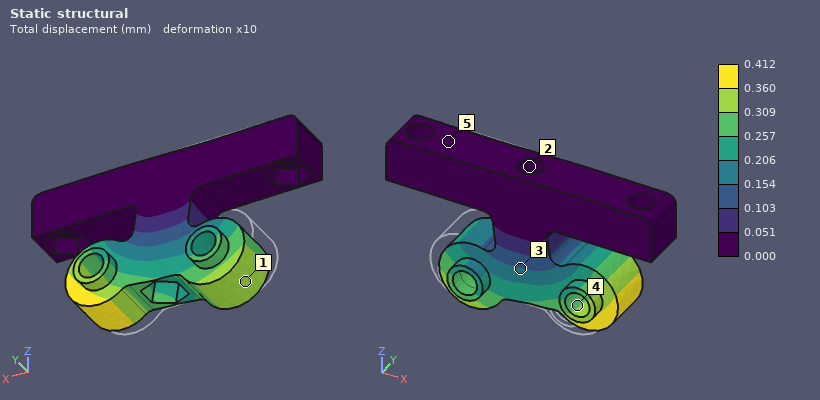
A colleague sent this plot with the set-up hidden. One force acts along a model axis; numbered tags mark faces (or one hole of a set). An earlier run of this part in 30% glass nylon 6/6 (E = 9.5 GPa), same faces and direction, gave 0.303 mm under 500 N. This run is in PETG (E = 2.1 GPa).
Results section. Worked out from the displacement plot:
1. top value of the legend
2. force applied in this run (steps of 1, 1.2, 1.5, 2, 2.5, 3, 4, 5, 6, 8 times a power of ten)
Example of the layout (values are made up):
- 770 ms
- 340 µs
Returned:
- 0.412 mm
- 150 N
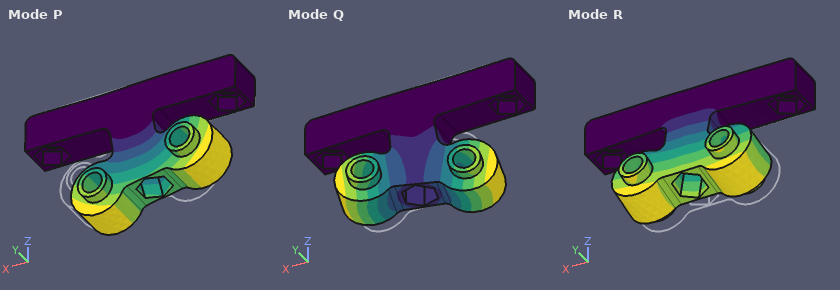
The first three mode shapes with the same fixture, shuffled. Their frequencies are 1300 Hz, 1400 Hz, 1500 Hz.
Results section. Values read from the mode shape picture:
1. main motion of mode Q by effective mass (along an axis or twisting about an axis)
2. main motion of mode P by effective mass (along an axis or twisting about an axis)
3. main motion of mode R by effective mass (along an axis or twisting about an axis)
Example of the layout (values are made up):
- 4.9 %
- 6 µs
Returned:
- twisting about Z
- along X
- along Y
